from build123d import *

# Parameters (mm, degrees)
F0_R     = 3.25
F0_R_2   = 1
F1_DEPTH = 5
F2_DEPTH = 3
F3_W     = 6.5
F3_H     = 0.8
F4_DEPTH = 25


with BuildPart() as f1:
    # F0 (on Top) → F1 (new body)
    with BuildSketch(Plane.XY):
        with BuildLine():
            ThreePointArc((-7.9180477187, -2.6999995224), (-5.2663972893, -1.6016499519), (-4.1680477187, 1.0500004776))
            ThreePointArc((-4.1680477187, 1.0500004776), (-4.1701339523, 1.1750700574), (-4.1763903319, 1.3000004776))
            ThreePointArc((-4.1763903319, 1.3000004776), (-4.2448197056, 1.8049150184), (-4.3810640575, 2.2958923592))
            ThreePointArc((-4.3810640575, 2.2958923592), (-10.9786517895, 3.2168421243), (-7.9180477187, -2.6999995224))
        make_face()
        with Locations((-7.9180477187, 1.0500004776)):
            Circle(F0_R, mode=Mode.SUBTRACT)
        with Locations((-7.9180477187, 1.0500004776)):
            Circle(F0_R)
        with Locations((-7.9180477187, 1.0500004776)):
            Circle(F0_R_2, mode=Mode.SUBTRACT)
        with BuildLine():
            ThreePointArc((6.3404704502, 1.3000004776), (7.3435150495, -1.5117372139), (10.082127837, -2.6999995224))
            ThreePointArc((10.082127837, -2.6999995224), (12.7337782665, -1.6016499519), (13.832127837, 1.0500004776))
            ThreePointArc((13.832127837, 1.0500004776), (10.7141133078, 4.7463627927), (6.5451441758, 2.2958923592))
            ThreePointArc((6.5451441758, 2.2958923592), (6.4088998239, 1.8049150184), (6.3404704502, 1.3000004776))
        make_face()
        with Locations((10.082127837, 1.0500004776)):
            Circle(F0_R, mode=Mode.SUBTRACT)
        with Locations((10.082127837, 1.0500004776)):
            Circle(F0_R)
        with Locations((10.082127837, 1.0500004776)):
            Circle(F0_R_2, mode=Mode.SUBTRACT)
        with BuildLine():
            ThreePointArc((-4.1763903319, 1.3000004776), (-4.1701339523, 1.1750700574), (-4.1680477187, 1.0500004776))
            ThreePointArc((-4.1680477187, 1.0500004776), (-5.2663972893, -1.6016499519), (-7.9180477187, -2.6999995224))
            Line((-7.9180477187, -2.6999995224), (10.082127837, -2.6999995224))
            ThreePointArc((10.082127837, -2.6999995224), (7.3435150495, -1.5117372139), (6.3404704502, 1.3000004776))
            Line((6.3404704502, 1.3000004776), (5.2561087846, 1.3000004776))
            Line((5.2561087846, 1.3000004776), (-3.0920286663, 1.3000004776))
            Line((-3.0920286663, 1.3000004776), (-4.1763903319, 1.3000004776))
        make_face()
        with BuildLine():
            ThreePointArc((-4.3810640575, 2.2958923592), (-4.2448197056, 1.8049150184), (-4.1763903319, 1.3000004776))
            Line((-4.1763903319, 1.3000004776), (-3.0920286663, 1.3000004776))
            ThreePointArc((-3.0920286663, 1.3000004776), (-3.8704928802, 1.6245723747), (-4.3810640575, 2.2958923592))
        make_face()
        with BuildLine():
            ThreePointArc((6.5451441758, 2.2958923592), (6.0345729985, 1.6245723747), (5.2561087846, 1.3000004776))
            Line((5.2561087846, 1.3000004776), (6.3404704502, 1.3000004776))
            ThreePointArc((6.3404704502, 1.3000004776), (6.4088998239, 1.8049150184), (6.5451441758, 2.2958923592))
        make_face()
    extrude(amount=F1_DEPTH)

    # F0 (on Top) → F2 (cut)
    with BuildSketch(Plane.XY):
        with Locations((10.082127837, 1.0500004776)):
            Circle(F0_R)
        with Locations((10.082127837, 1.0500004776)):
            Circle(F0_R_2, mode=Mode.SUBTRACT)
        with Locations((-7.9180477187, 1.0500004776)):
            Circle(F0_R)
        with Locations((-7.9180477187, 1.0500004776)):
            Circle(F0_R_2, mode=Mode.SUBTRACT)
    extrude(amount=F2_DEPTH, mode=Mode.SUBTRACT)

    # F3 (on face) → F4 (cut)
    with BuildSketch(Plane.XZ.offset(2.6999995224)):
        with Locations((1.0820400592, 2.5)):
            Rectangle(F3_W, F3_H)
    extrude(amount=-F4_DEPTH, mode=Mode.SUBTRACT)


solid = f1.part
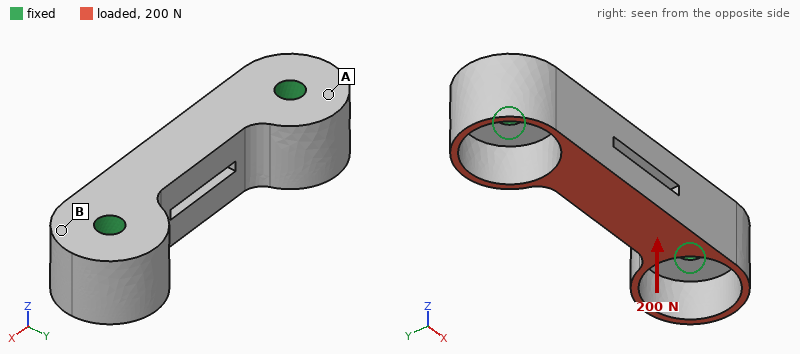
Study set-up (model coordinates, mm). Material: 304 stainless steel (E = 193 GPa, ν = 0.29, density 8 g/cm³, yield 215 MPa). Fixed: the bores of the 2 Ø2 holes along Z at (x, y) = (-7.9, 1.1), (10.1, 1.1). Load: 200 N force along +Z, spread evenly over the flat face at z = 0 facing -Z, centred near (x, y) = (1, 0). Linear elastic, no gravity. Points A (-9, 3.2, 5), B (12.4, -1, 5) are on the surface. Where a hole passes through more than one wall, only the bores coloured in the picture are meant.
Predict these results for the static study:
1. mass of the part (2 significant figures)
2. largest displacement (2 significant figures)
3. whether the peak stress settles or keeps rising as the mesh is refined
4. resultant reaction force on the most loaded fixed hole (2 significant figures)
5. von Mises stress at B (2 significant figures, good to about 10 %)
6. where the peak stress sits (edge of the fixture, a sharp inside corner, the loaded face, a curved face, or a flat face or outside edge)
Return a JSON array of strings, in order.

["3.6 g", "2.2 µm", "keeps rising", "110 N", "9.7 MPa", "edge of the fixture"]
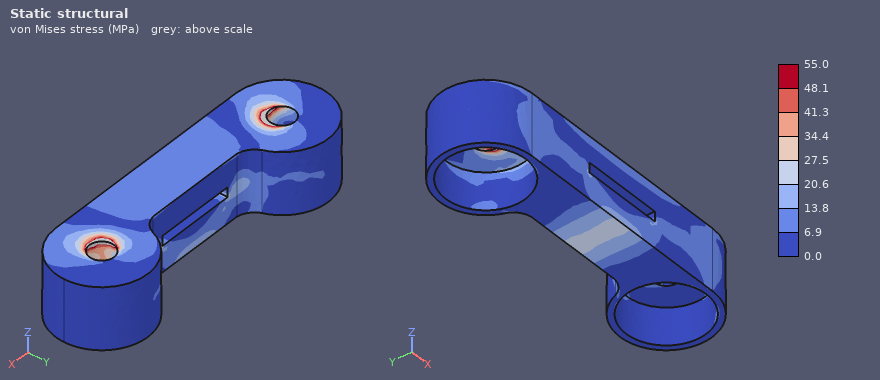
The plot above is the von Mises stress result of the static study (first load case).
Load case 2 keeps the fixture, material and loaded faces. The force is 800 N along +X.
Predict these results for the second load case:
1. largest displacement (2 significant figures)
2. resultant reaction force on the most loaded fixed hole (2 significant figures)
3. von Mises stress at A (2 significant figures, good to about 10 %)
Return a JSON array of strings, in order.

["4.0 µm", "430 N", "16 MPa"]
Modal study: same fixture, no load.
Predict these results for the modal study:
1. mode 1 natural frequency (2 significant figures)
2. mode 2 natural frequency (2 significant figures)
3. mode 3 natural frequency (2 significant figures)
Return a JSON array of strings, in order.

["32 kHz", "46 kHz", "59 kHz"]
